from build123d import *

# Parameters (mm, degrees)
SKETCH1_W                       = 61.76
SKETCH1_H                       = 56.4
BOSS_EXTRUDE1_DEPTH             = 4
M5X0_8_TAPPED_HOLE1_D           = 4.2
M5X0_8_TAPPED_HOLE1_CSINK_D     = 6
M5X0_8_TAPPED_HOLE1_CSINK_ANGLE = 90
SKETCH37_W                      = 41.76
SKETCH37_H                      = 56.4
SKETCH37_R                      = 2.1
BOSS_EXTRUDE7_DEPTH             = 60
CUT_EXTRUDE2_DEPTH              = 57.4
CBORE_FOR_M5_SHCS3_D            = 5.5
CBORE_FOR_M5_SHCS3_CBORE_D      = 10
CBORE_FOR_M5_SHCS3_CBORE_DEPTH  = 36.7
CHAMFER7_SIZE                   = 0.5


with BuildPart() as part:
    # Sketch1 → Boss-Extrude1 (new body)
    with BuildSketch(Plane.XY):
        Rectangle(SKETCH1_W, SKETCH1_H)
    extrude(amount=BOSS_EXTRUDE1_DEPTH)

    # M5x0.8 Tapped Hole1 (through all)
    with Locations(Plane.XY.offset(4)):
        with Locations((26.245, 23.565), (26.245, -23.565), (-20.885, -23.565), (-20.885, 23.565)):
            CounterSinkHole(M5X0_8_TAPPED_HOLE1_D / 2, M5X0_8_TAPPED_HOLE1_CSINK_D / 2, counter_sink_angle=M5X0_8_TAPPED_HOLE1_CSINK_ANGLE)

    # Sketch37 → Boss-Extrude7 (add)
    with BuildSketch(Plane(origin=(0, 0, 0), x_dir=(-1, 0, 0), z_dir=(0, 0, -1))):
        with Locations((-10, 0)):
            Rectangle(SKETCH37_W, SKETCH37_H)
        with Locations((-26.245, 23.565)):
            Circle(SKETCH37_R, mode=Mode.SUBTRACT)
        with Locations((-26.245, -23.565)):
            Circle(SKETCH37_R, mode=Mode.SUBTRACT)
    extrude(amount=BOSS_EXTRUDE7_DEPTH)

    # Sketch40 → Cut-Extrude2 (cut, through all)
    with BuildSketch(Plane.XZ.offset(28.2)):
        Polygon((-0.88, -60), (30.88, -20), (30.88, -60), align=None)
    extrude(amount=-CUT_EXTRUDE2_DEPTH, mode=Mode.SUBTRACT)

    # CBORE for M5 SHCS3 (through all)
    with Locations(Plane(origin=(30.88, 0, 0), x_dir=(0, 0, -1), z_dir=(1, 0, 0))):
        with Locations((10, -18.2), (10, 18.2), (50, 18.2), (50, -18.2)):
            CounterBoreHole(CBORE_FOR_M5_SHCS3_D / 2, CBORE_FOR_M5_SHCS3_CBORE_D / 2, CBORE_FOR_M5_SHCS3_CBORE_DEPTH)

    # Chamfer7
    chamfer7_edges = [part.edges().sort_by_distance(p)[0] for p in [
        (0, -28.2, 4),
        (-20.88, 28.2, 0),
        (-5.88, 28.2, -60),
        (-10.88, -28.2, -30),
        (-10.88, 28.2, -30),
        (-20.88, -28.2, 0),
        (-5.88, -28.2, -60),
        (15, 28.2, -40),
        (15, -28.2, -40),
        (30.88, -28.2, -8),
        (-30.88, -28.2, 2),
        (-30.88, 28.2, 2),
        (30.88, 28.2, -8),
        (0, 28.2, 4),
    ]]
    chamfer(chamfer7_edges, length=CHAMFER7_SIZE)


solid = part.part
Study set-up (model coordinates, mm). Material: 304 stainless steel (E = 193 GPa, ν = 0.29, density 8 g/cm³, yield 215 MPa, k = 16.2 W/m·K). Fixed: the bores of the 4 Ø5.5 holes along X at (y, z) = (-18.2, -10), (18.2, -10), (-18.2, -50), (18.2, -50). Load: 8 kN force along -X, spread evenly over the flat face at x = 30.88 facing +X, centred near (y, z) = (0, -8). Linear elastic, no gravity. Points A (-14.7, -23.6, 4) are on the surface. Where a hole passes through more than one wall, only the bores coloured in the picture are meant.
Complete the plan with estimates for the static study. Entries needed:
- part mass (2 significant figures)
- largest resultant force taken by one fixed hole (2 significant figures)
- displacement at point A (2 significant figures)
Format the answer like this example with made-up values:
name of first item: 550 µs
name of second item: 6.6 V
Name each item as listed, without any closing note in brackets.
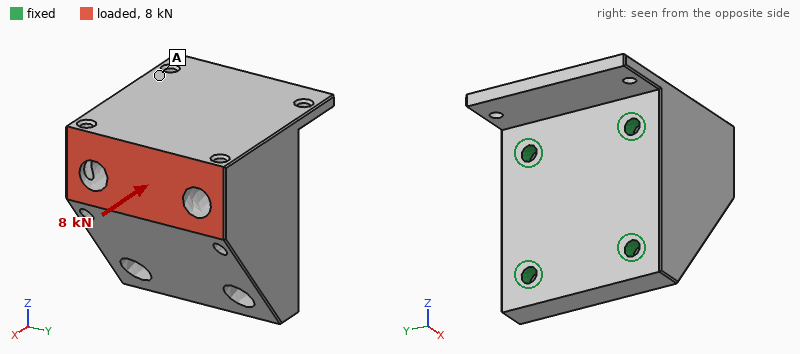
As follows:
part mass: 880 g
largest resultant force taken by one fixed hole: 4.2 kN
displacement at point A: 4.3 µm
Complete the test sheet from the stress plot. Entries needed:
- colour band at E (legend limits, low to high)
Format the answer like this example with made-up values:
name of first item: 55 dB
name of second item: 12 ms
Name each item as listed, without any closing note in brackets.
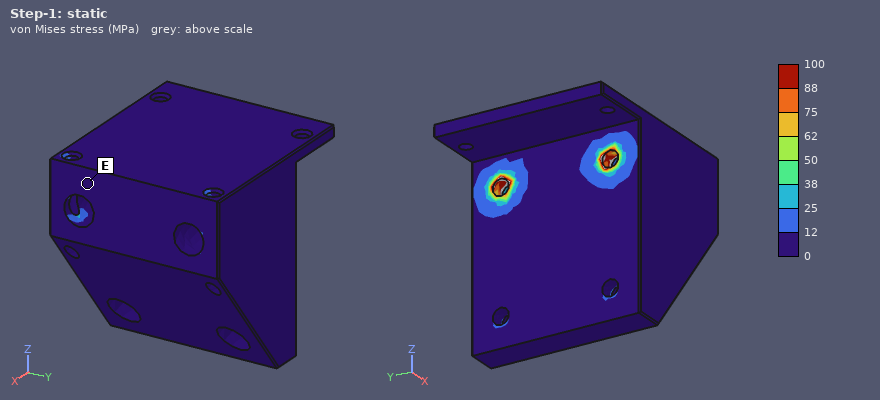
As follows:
colour band at E: 0 to 12 MPa
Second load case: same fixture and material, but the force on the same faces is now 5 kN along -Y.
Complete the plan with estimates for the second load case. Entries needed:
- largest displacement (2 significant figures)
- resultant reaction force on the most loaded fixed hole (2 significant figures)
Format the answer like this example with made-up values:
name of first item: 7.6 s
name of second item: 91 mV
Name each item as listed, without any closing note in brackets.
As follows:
largest displacement: 9.3 µm
resultant reaction force on the most loaded fixed hole: 3.7 kN
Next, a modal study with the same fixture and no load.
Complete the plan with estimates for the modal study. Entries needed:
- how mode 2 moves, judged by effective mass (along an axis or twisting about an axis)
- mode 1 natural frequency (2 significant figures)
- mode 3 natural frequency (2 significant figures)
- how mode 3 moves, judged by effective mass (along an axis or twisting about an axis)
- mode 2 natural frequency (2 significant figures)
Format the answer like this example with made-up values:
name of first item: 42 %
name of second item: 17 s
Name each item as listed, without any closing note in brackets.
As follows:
how mode 2 moves, judged by effective mass: along Y
mode 1 natural frequency: 6300 Hz
mode 3 natural frequency: 8500 Hz
how mode 3 moves, judged by effective mass: along Z
mode 2 natural frequency: 8200 Hz
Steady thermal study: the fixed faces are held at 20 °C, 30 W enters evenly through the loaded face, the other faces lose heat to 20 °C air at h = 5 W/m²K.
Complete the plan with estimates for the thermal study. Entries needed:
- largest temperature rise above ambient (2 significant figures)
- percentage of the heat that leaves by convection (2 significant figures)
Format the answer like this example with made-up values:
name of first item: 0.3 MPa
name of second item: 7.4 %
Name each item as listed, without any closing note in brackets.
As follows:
largest temperature rise above ambient: 65 K
percentage of the heat that leaves by convection: 8.2 %
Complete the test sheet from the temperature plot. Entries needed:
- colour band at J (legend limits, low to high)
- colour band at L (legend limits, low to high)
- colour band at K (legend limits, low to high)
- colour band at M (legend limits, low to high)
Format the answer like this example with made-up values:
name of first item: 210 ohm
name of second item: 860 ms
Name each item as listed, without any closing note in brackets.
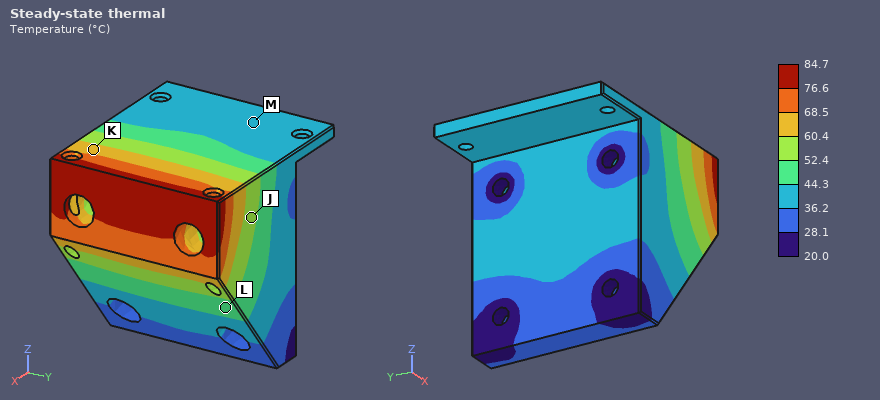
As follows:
colour band at J: 52.4 to 60.4 °C
colour band at L: 44.3 to 52.4 °C
colour band at K: 60.4 to 68.5 °C
colour band at M: 36.2 to 44.3 °C
